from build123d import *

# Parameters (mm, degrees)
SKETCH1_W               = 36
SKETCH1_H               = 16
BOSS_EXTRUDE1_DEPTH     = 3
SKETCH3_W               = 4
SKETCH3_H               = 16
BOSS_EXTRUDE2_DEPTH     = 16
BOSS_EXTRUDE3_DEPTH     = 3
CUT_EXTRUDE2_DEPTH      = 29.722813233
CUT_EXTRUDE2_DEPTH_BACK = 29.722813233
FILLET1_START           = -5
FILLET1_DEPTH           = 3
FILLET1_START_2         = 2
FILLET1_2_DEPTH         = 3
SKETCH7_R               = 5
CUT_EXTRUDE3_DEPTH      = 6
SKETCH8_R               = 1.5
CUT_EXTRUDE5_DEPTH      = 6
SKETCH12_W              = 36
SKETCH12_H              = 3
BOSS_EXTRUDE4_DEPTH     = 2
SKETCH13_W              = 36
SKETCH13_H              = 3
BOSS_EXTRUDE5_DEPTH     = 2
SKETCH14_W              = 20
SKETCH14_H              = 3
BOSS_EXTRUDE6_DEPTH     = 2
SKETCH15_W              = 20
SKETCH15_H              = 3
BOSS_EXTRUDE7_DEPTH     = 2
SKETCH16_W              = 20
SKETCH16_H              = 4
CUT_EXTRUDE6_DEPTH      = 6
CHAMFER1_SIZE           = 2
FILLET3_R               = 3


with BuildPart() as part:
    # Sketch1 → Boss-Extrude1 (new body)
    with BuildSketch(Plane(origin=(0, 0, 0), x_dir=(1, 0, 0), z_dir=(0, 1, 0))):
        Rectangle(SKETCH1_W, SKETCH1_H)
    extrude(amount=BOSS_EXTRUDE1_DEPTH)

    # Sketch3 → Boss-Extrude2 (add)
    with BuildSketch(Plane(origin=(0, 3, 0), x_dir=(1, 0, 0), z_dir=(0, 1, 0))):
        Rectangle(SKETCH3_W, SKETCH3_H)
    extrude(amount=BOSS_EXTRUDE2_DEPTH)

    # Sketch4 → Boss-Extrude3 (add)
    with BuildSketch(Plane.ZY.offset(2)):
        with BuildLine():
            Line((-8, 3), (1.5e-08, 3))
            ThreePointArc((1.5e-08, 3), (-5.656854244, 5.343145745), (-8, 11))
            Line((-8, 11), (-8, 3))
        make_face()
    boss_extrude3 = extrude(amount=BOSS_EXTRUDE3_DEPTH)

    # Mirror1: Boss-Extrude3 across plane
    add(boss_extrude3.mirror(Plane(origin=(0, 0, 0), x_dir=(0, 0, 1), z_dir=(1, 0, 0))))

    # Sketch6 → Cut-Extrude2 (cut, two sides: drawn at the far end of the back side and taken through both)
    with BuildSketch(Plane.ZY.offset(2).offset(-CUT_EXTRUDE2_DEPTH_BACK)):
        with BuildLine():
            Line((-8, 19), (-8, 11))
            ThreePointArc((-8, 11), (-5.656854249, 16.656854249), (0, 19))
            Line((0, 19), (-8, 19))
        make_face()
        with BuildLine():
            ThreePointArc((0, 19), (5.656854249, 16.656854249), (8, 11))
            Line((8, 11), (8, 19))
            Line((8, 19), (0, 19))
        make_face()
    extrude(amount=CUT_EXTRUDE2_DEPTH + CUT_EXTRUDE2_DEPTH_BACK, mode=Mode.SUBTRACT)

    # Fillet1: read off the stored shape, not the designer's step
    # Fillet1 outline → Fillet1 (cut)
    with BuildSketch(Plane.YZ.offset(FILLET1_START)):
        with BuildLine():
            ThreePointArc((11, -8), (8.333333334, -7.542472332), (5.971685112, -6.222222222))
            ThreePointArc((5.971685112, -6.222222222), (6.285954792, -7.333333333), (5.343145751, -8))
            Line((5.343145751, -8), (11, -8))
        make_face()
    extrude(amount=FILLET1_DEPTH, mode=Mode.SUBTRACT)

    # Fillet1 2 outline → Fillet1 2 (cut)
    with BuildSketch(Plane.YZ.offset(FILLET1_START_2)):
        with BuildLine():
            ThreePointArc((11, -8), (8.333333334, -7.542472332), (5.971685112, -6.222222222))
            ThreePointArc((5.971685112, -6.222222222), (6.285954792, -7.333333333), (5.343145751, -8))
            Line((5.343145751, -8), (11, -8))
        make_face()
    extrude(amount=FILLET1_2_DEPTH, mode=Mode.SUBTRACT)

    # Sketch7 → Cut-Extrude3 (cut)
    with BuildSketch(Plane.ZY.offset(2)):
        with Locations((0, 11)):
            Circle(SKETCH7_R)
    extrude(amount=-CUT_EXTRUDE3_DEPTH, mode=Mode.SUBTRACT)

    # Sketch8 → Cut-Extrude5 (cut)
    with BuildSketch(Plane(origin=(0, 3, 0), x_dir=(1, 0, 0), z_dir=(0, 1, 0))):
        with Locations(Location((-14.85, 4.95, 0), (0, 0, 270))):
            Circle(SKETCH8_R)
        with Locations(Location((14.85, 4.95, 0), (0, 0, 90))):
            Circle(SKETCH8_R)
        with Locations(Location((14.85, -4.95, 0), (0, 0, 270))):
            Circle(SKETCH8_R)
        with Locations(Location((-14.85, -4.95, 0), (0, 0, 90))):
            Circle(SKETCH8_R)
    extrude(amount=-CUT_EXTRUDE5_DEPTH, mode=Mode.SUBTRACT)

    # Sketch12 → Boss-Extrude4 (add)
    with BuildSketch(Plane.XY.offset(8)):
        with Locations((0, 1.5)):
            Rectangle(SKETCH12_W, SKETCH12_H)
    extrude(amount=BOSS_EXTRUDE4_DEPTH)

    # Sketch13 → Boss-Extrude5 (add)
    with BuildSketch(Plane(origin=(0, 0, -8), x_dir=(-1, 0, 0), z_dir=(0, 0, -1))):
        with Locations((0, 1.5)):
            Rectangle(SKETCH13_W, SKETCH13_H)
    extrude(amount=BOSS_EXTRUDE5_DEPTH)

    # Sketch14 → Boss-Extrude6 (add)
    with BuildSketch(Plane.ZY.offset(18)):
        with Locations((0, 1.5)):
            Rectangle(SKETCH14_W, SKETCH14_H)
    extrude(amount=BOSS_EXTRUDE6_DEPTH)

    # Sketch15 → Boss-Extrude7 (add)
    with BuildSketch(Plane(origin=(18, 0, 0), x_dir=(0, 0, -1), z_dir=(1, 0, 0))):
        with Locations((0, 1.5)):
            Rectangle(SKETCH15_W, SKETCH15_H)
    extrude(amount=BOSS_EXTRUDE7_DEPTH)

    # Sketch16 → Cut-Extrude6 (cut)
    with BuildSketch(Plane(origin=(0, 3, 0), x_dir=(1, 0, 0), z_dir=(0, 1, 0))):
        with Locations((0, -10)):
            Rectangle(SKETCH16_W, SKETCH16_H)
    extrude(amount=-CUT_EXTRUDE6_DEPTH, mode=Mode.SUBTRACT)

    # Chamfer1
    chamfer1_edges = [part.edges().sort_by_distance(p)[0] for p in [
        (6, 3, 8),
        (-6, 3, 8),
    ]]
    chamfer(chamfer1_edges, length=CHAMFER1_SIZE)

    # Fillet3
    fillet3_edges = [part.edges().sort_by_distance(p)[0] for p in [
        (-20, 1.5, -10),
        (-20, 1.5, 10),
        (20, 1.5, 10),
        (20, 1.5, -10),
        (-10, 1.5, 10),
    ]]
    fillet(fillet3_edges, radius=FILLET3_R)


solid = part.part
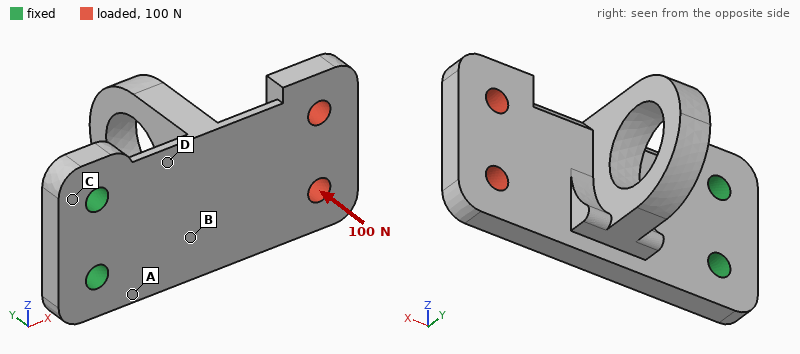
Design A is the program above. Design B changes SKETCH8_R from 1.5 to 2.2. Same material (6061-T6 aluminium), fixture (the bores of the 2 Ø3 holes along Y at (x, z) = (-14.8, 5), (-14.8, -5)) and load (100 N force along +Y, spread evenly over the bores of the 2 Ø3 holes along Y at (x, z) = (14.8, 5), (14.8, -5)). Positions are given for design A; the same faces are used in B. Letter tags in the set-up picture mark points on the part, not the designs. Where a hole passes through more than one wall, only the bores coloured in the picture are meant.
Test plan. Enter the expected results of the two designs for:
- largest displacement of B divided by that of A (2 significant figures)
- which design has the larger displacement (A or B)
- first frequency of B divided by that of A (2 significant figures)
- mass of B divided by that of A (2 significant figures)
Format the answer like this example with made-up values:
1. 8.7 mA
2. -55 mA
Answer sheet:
1. 0.91
2. A
3. 1.1
4. 0.97
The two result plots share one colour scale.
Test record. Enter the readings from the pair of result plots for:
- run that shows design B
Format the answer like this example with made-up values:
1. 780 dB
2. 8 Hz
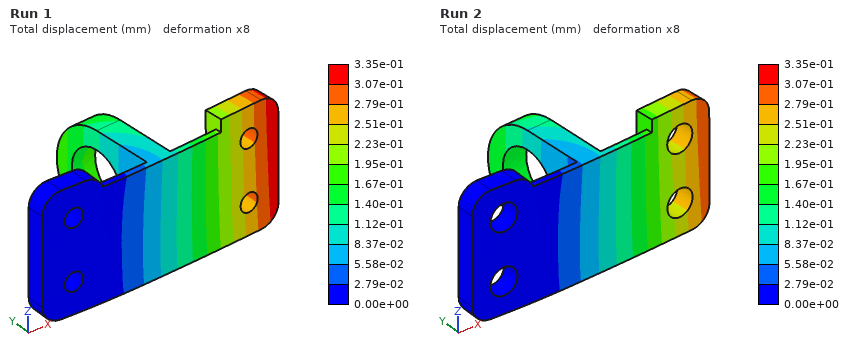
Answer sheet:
1. Run 2
